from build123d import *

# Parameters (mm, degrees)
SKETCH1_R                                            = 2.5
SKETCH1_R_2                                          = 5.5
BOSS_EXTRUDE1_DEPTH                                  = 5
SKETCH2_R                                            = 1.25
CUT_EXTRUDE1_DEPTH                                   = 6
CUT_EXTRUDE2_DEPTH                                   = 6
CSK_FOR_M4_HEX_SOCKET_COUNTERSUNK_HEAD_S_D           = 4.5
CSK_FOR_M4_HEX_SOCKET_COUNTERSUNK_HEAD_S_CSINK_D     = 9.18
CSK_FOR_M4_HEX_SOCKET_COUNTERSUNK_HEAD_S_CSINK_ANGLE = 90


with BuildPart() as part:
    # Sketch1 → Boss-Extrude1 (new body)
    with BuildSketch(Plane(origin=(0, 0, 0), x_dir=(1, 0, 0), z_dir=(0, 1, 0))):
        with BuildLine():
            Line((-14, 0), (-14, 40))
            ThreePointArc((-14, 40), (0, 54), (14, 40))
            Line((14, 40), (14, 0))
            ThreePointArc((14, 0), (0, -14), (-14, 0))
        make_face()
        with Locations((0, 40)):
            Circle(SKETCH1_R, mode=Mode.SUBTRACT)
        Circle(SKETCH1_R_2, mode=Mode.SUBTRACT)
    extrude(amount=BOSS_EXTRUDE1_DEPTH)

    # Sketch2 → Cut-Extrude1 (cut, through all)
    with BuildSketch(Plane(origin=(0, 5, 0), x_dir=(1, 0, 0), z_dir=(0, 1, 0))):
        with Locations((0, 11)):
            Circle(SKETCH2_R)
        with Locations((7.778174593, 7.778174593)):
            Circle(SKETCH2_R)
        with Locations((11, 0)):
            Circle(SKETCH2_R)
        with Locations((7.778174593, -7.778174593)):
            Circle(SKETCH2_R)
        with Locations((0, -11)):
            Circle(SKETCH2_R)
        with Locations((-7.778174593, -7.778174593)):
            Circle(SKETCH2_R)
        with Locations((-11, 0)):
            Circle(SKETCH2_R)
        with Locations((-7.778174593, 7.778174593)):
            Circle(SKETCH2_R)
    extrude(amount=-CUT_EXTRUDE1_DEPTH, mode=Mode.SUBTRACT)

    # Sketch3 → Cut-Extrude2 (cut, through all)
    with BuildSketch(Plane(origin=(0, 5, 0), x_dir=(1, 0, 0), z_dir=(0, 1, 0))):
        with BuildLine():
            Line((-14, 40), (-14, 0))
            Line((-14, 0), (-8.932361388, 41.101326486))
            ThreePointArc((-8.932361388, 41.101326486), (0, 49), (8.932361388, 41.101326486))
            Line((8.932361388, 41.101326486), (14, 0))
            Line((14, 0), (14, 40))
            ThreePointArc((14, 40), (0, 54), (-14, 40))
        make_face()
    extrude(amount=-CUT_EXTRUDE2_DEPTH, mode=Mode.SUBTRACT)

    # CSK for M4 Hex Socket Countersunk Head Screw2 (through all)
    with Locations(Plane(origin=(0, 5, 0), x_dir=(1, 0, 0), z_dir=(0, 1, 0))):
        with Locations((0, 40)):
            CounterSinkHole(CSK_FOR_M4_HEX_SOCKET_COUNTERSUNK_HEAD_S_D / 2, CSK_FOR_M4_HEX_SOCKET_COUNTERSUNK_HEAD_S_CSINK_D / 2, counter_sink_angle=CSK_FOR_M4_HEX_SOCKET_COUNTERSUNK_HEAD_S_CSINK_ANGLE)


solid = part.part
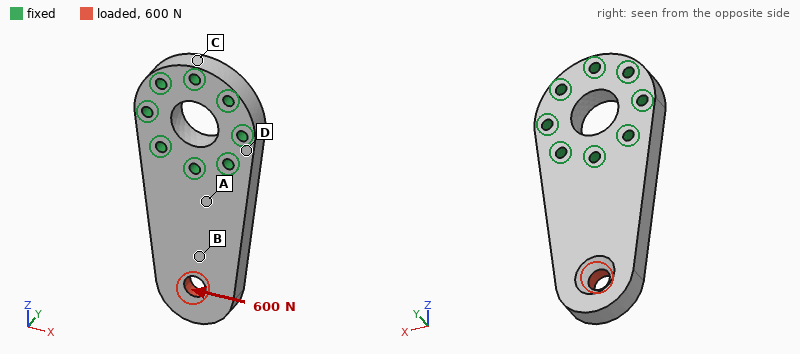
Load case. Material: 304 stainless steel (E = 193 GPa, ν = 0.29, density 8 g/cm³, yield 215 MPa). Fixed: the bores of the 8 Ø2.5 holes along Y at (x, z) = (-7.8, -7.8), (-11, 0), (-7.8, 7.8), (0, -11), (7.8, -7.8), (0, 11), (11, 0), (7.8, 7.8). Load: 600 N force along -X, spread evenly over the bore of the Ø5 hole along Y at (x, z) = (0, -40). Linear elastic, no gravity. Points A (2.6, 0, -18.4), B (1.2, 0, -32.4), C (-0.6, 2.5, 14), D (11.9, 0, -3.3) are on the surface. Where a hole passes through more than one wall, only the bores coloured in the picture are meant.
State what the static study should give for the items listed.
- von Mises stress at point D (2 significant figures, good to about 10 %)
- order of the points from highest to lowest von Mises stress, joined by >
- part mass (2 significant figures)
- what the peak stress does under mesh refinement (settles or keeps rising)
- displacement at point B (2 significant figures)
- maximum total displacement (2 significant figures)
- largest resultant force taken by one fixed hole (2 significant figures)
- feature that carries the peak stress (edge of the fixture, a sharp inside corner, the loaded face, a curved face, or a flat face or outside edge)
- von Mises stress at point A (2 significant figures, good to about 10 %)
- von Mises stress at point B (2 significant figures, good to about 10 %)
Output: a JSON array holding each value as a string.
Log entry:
["10 MPa", "B > A > D > C", "48 g", "keeps rising", "6.2 µm", "13 µm", "790 N", "edge of the fixture", "17 MPa", "22 MPa"]
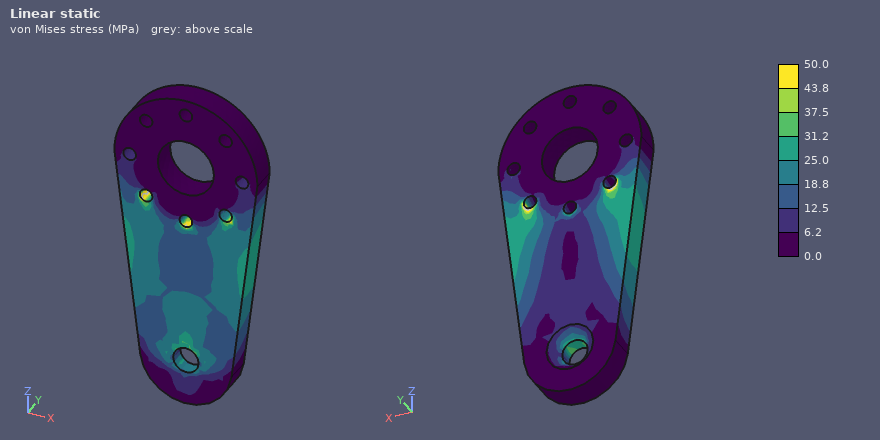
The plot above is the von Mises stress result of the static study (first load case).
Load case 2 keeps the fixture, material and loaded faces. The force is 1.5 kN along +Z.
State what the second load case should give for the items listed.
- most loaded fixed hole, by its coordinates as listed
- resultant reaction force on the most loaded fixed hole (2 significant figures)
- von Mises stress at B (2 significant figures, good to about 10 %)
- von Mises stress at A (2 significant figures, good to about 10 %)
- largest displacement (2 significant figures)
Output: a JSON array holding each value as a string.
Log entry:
["(0, -11)", "590 N", "37 MPa", "30 MPa", "26 µm"]
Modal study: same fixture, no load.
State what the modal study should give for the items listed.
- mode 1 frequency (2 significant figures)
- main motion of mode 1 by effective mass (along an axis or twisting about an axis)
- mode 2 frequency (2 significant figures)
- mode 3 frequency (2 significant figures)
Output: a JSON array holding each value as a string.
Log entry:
["3300 Hz", "along Y", "12 kHz", "12 kHz"]
